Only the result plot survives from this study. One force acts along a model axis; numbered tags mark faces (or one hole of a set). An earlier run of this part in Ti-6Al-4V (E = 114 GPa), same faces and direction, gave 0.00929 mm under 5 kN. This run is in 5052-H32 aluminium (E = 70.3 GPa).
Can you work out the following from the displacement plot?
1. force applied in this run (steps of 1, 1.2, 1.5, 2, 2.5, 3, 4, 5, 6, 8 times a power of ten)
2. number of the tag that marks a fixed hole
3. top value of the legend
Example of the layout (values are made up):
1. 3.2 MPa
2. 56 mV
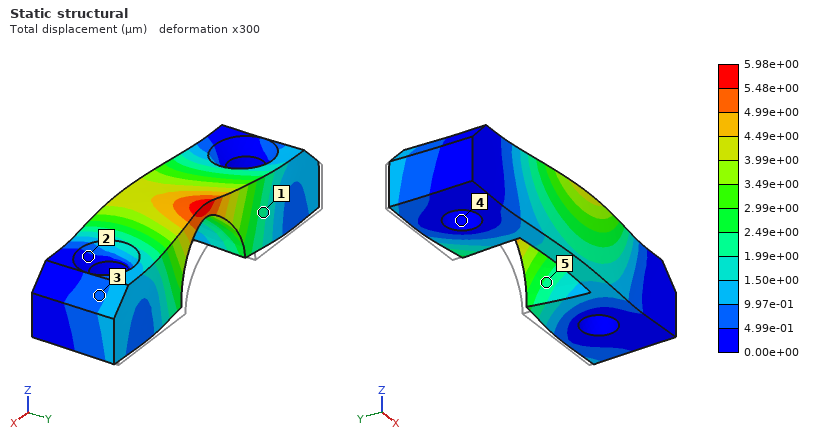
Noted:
1. 2 kN
2. 4
3. 5.98e+00 µm
